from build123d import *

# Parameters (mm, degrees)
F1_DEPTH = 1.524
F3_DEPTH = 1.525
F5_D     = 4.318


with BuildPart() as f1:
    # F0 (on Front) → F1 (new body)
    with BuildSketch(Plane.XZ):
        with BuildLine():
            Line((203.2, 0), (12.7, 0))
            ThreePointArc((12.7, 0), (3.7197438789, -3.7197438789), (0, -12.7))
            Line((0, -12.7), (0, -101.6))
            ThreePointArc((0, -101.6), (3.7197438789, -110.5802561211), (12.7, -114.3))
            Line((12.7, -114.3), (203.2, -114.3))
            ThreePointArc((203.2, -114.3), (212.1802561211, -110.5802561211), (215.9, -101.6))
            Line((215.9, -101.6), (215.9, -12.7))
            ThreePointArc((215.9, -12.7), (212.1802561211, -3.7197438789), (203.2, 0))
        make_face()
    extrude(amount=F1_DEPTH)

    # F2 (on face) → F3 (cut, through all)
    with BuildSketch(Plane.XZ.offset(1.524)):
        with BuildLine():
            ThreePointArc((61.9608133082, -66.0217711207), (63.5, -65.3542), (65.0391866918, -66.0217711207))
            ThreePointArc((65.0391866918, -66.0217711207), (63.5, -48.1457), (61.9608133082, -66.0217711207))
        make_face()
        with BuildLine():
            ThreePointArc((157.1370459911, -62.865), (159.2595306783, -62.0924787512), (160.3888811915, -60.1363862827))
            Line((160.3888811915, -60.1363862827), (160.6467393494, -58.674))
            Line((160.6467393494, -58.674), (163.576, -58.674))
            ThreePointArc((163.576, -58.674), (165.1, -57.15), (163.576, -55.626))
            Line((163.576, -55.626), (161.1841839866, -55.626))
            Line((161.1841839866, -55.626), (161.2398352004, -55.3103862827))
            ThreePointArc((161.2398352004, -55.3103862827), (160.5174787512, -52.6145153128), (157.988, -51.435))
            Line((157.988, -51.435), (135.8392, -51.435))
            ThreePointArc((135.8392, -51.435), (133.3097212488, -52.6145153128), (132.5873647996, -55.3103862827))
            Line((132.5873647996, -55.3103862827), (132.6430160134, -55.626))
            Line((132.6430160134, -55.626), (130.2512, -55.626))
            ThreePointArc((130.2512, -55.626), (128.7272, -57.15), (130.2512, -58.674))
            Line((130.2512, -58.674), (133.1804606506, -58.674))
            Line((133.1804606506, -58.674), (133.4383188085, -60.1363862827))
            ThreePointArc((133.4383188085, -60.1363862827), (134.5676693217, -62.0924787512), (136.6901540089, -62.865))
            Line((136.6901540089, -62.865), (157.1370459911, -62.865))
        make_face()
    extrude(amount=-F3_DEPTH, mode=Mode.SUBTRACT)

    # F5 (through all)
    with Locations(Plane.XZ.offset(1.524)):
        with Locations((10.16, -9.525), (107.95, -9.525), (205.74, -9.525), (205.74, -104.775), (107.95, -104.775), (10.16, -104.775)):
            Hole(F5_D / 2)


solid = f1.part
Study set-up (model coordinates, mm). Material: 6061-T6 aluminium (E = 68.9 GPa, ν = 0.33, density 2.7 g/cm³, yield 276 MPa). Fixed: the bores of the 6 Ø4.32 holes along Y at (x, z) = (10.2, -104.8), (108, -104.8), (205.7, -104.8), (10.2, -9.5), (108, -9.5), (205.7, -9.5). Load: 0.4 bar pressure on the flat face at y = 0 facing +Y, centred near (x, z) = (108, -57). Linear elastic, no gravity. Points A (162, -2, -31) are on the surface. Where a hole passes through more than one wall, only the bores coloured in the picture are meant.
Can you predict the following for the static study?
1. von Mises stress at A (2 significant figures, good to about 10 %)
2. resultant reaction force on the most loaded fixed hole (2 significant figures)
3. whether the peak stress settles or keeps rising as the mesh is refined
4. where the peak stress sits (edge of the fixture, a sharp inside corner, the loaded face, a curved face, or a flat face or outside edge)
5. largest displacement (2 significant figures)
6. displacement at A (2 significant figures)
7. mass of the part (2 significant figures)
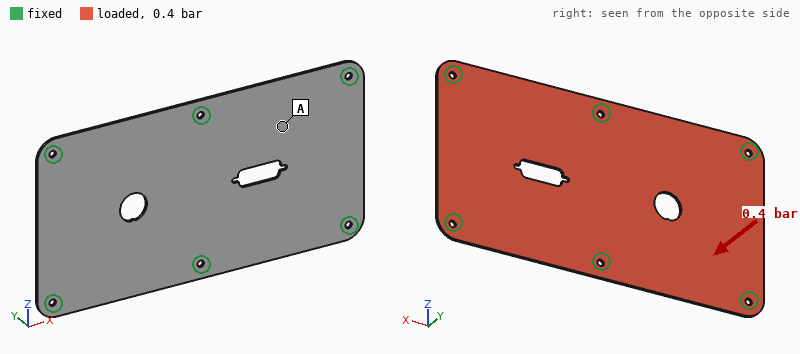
41 MPa
230 N
keeps rising
edge of the fixture
1.2 mm
0.87 mm
98 g
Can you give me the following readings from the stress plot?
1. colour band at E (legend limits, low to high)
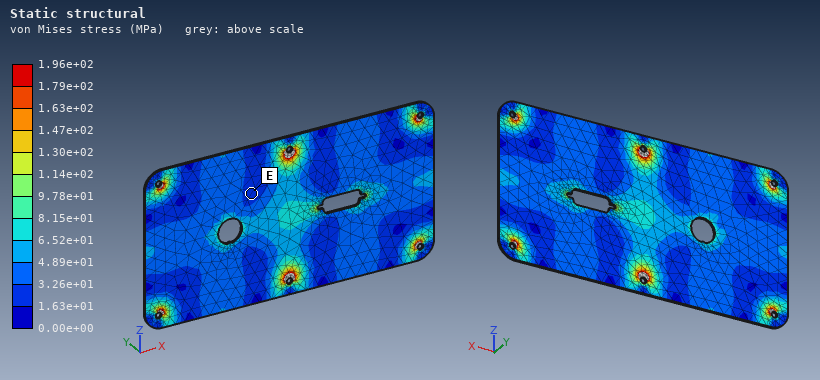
1.63e+01 to 3.26e+01 MPa
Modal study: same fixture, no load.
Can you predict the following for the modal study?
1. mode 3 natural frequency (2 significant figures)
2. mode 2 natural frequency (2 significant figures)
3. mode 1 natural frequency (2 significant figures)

920 Hz
580 Hz
570 Hz
